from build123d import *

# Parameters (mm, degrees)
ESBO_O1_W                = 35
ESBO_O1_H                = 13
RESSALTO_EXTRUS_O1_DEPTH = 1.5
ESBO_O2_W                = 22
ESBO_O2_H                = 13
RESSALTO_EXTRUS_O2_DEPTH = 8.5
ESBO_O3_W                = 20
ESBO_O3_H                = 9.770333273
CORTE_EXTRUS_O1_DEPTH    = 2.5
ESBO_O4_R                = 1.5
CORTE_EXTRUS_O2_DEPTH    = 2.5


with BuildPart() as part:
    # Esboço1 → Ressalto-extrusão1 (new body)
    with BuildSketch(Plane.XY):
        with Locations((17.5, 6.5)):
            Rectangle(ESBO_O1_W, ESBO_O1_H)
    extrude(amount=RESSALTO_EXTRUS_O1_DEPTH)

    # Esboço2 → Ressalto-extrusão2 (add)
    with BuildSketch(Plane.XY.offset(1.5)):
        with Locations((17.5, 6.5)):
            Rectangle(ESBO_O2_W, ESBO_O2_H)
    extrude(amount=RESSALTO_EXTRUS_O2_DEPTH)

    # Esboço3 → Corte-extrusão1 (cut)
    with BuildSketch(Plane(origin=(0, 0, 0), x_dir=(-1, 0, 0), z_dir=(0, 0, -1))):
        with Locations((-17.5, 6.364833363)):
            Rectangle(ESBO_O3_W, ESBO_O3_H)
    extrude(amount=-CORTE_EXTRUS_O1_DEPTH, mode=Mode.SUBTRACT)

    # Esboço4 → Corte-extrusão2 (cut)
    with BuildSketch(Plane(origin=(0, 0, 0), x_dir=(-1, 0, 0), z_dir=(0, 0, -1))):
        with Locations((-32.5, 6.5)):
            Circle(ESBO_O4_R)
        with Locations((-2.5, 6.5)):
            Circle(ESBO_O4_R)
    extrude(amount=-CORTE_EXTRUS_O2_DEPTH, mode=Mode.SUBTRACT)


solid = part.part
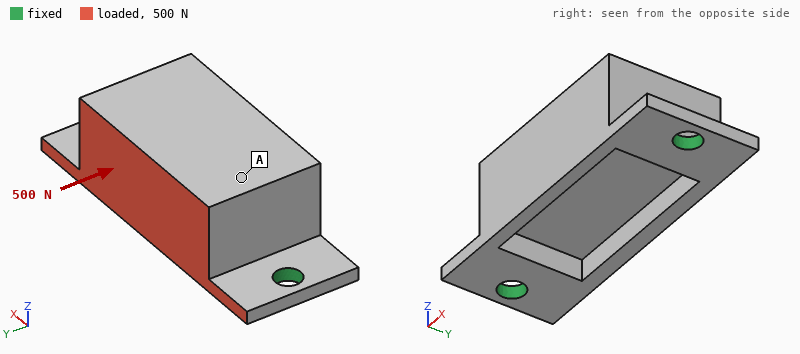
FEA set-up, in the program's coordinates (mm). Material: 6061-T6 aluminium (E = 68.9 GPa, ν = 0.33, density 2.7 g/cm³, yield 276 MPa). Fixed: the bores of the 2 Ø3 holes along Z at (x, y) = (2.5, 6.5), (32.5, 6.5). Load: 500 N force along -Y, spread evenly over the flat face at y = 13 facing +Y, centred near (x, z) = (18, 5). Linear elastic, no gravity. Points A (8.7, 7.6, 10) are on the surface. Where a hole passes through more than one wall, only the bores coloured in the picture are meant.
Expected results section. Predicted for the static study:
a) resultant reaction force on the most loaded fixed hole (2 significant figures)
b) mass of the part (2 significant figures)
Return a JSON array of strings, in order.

["250 N", "7.0 g"]
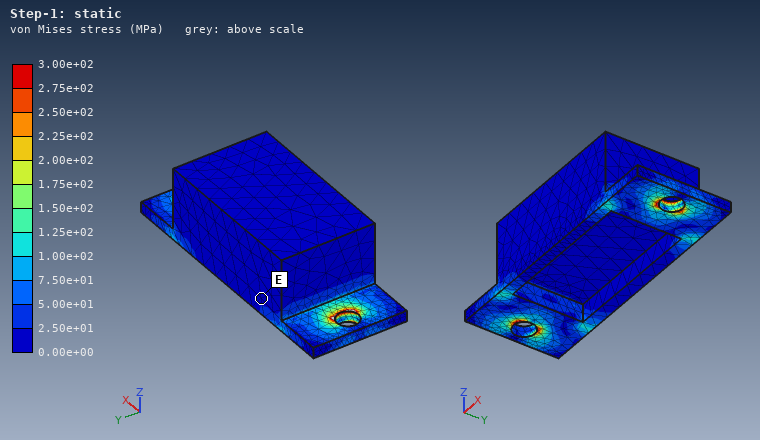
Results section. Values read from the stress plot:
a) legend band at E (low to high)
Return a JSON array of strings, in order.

["0.00e+00 to 2.50e+01 MPa"]
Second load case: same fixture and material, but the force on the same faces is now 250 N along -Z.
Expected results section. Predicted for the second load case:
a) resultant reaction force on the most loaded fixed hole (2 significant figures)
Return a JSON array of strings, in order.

["150 N"]
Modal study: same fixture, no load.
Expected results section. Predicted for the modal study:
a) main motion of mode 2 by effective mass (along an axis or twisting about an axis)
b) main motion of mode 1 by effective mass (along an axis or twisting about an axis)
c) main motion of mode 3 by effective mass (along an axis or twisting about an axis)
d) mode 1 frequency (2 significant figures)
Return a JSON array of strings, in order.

["along Z", "along Y", "along X", "4700 Hz"]
